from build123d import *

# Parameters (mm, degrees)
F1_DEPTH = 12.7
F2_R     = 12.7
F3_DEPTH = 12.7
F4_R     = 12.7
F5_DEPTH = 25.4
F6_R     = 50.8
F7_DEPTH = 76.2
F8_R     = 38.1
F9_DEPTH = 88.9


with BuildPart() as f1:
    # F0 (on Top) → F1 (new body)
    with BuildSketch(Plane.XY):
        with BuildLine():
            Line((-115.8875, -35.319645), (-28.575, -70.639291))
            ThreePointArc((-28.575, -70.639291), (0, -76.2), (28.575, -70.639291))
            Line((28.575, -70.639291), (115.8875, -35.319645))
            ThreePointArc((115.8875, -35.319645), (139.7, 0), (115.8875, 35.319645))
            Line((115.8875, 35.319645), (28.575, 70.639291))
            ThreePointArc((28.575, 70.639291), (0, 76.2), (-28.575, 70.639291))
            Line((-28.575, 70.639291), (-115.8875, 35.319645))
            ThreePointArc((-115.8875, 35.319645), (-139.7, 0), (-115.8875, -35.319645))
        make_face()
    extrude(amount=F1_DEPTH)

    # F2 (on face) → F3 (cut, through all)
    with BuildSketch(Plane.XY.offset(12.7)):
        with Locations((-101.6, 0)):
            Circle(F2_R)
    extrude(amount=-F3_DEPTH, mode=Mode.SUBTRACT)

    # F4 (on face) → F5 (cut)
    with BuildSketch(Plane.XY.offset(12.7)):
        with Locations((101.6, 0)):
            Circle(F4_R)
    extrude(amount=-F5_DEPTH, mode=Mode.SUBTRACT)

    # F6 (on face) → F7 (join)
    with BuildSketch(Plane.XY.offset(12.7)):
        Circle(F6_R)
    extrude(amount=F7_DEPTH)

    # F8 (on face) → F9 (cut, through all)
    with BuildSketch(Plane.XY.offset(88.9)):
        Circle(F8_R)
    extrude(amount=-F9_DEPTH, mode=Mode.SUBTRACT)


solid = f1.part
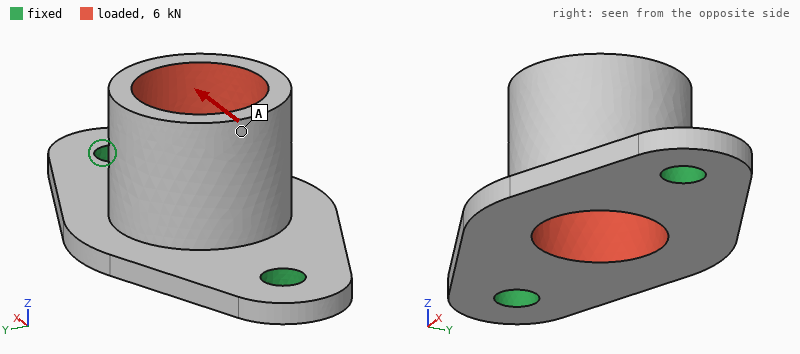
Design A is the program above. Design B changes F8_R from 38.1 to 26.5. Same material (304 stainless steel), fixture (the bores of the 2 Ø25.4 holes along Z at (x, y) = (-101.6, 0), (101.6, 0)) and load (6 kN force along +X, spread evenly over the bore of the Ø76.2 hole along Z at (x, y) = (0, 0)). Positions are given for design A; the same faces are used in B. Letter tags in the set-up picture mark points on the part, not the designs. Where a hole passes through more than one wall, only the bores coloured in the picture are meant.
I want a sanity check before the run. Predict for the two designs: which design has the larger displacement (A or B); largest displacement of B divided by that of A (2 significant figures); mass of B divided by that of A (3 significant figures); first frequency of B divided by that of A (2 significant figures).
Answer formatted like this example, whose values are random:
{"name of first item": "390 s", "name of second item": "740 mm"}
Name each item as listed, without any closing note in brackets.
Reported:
{"which design has the larger displacement": "A", "largest displacement of B divided by that of A": "0.85", "mass of B divided by that of A": "1.37", "first frequency of B divided by that of A": "0.86"}
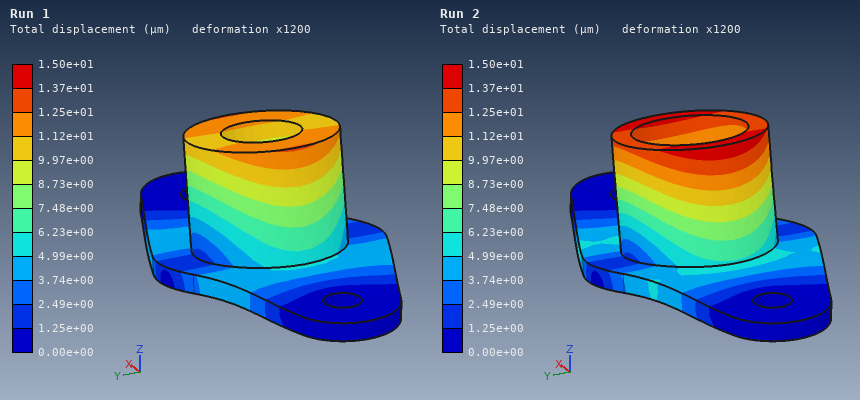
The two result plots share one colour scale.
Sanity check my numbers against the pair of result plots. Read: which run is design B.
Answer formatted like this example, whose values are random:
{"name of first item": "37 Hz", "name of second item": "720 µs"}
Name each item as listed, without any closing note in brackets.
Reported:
{"which run is design B": "Run 1"}
